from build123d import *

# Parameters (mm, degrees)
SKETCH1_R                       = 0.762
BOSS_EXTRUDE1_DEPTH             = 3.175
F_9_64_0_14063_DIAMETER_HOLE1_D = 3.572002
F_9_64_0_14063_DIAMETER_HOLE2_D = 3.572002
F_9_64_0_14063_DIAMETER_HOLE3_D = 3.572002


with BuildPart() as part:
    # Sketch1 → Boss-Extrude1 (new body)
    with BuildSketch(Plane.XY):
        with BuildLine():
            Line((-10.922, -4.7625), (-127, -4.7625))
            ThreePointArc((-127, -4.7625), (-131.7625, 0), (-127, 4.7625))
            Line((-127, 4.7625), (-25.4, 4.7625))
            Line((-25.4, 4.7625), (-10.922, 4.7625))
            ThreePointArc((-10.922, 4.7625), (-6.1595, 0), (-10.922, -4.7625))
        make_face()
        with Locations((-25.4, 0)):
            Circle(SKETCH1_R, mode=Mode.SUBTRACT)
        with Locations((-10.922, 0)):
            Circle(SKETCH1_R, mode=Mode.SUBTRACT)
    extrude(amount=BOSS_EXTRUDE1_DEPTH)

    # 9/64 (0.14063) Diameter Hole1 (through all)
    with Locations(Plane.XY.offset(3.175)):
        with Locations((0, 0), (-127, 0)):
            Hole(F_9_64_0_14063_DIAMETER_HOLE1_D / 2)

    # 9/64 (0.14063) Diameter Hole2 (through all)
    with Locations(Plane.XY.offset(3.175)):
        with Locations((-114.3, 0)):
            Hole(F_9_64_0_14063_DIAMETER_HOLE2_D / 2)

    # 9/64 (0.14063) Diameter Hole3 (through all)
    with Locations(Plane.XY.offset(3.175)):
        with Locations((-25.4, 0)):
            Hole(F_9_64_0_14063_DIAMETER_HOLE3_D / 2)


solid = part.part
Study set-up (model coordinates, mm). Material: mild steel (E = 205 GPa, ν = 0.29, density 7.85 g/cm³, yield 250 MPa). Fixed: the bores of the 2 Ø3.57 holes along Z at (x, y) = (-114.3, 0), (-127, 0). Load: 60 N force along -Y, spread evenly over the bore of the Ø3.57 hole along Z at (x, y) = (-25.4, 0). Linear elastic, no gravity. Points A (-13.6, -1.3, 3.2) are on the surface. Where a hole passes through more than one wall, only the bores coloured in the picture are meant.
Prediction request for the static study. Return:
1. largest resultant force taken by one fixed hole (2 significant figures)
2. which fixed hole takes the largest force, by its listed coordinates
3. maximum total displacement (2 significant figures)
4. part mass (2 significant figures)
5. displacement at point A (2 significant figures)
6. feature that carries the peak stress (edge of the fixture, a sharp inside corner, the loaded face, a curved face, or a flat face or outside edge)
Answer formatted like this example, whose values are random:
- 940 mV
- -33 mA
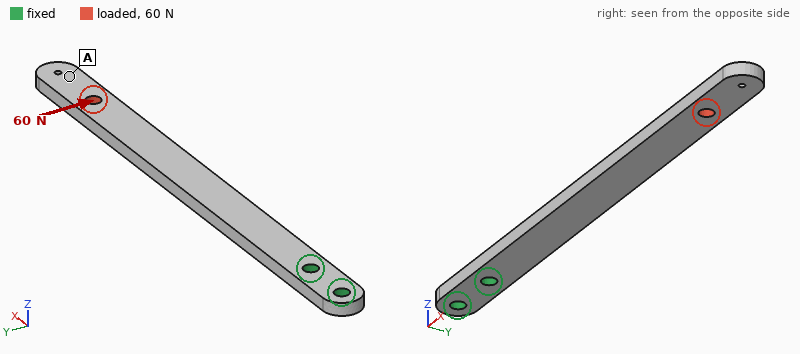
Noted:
- 220 N
- (-114.3, 0)
- 0.42 mm
- 29 g
- 0.38 mm
- edge of the fixture
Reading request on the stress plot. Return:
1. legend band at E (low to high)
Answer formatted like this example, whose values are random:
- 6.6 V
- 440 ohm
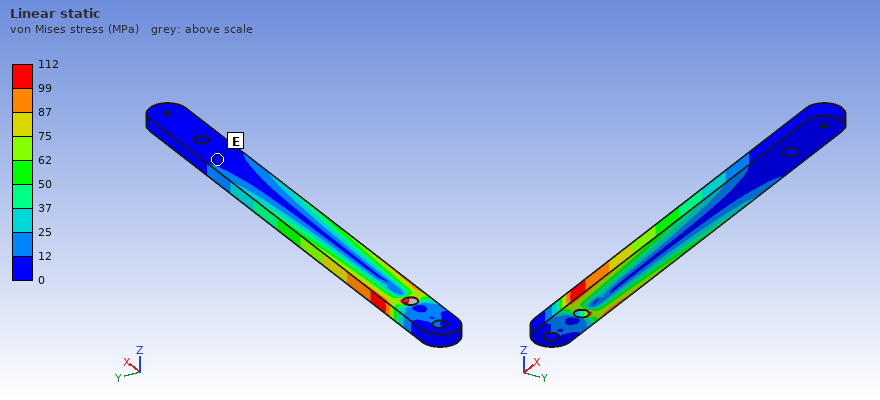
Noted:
- 0 to 12 MPa
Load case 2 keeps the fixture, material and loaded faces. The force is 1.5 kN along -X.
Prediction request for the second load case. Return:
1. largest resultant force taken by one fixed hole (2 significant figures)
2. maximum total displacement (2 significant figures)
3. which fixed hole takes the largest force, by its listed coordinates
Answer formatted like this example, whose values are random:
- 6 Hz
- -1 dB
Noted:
- 1.4 kN
- 23 µm
- (-114.3, 0)
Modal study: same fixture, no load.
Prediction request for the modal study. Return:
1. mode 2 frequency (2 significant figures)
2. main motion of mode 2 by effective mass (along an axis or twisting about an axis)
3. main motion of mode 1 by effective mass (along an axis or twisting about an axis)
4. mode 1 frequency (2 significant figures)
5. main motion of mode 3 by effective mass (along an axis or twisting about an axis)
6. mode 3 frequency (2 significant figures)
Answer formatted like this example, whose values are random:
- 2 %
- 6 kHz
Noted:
- 670 Hz
- along Y
- along Z
- 240 Hz
- along Z
- 1500 Hz
